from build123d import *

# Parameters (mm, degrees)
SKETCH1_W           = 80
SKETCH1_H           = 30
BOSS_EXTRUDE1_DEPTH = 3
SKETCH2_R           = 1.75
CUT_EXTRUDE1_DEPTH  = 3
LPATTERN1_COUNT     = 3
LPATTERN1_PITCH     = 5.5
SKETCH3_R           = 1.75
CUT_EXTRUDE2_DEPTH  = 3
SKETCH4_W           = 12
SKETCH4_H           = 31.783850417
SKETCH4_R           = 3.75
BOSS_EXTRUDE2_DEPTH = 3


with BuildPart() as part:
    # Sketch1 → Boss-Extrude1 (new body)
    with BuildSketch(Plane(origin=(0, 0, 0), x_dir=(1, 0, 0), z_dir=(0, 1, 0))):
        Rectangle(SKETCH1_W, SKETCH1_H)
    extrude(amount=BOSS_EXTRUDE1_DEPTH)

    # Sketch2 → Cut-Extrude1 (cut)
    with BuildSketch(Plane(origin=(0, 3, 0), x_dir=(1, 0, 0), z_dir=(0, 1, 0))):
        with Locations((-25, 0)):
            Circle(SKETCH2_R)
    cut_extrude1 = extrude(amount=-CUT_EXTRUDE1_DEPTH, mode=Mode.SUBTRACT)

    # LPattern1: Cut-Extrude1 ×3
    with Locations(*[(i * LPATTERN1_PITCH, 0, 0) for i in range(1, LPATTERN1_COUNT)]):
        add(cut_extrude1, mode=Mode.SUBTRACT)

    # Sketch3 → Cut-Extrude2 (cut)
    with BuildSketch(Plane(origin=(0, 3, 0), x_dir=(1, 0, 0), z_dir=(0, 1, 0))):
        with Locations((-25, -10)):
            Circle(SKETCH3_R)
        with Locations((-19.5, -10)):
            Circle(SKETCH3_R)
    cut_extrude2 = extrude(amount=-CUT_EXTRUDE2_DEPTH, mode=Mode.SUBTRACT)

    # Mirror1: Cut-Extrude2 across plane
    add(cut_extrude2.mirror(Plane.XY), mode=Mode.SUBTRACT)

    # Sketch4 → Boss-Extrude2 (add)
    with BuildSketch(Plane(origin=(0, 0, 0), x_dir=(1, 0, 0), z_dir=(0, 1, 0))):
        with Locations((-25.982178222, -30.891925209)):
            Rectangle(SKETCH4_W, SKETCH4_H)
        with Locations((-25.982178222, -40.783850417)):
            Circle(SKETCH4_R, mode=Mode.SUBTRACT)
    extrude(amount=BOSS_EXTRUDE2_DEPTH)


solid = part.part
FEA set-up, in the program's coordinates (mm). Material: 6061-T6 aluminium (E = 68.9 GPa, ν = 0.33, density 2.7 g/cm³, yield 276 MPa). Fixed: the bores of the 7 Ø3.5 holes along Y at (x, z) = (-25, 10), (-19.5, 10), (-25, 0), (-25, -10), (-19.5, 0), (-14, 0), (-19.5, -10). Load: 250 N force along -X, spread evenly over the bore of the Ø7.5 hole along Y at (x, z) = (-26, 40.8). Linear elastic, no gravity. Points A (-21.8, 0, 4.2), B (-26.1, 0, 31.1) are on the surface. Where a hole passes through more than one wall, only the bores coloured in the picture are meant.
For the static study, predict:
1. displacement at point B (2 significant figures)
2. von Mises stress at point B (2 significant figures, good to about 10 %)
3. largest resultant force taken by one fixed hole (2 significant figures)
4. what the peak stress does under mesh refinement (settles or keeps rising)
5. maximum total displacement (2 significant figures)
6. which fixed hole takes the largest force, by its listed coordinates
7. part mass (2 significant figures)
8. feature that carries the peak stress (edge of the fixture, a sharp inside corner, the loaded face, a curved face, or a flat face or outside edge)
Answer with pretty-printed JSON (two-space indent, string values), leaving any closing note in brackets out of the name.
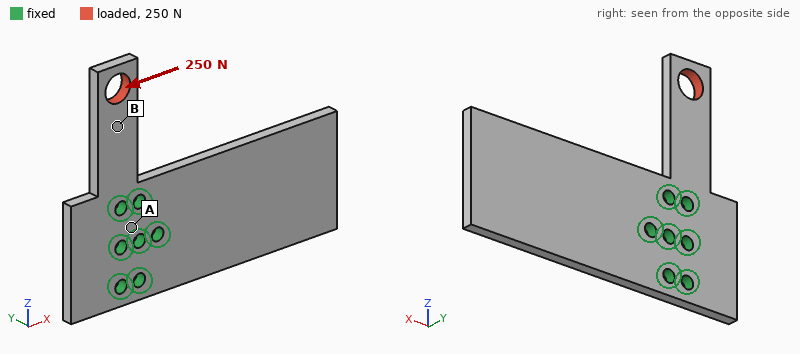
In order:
{
  "displacement at point B": "0.043 mm",
  "von Mises stress at point B": "21 MPa",
  "largest resultant force taken by one fixed hole": "640 N",
  "what the peak stress does under mesh refinement": "keeps rising",
  "maximum total displacement": "0.11 mm",
  "which fixed hole takes the largest force, by its listed coordinates": "(-19.5, 10)",
  "part mass": "22 g",
  "feature that carries the peak stress": "a sharp inside corner"
}
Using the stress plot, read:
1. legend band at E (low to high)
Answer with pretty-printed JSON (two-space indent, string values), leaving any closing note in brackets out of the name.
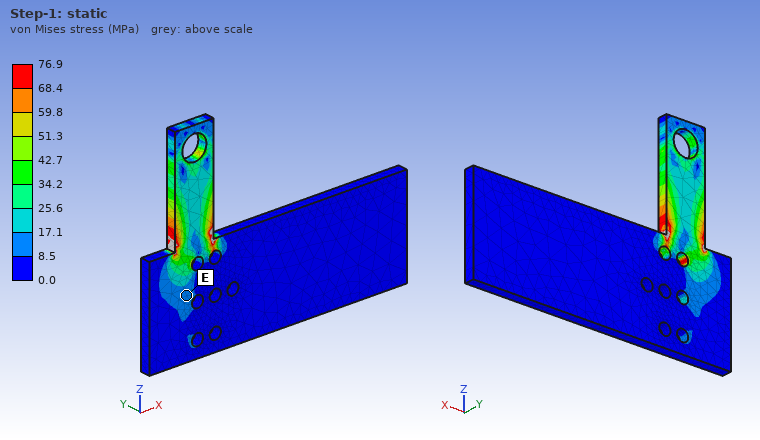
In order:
{
  "legend band at E": "8.5 to 17.1 MPa"
}
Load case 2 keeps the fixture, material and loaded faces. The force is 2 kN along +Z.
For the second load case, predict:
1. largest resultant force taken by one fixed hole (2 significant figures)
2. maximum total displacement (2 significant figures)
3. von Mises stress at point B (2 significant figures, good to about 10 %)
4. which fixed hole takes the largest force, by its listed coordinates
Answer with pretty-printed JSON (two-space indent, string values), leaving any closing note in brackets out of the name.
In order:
{
  "largest resultant force taken by one fixed hole": "1.4 kN",
  "maximum total displacement": "47 µm",
  "von Mises stress at point B": "40 MPa",
  "which fixed hole takes the largest force, by its listed coordinates": "(-25, 10)"
}
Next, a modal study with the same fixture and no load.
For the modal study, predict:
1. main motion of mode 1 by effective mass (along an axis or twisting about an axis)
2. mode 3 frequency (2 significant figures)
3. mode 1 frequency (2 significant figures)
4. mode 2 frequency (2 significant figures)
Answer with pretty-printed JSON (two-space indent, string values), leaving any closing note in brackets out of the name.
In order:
{
  "main motion of mode 1 by effective mass": "along Y",
  "mode 3 frequency": "3000 Hz",
  "mode 1 frequency": "840 Hz",
  "mode 2 frequency": "2300 Hz"
}
